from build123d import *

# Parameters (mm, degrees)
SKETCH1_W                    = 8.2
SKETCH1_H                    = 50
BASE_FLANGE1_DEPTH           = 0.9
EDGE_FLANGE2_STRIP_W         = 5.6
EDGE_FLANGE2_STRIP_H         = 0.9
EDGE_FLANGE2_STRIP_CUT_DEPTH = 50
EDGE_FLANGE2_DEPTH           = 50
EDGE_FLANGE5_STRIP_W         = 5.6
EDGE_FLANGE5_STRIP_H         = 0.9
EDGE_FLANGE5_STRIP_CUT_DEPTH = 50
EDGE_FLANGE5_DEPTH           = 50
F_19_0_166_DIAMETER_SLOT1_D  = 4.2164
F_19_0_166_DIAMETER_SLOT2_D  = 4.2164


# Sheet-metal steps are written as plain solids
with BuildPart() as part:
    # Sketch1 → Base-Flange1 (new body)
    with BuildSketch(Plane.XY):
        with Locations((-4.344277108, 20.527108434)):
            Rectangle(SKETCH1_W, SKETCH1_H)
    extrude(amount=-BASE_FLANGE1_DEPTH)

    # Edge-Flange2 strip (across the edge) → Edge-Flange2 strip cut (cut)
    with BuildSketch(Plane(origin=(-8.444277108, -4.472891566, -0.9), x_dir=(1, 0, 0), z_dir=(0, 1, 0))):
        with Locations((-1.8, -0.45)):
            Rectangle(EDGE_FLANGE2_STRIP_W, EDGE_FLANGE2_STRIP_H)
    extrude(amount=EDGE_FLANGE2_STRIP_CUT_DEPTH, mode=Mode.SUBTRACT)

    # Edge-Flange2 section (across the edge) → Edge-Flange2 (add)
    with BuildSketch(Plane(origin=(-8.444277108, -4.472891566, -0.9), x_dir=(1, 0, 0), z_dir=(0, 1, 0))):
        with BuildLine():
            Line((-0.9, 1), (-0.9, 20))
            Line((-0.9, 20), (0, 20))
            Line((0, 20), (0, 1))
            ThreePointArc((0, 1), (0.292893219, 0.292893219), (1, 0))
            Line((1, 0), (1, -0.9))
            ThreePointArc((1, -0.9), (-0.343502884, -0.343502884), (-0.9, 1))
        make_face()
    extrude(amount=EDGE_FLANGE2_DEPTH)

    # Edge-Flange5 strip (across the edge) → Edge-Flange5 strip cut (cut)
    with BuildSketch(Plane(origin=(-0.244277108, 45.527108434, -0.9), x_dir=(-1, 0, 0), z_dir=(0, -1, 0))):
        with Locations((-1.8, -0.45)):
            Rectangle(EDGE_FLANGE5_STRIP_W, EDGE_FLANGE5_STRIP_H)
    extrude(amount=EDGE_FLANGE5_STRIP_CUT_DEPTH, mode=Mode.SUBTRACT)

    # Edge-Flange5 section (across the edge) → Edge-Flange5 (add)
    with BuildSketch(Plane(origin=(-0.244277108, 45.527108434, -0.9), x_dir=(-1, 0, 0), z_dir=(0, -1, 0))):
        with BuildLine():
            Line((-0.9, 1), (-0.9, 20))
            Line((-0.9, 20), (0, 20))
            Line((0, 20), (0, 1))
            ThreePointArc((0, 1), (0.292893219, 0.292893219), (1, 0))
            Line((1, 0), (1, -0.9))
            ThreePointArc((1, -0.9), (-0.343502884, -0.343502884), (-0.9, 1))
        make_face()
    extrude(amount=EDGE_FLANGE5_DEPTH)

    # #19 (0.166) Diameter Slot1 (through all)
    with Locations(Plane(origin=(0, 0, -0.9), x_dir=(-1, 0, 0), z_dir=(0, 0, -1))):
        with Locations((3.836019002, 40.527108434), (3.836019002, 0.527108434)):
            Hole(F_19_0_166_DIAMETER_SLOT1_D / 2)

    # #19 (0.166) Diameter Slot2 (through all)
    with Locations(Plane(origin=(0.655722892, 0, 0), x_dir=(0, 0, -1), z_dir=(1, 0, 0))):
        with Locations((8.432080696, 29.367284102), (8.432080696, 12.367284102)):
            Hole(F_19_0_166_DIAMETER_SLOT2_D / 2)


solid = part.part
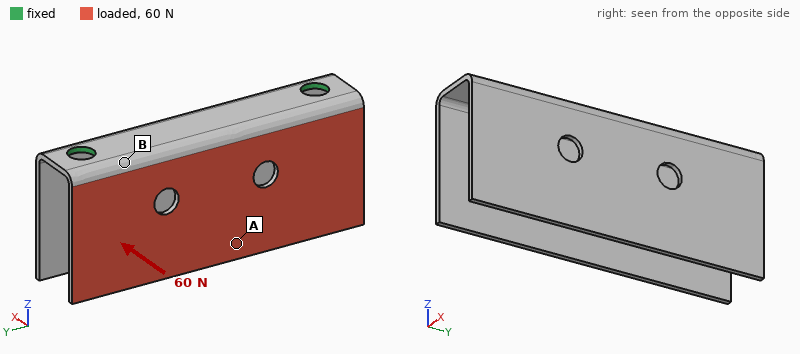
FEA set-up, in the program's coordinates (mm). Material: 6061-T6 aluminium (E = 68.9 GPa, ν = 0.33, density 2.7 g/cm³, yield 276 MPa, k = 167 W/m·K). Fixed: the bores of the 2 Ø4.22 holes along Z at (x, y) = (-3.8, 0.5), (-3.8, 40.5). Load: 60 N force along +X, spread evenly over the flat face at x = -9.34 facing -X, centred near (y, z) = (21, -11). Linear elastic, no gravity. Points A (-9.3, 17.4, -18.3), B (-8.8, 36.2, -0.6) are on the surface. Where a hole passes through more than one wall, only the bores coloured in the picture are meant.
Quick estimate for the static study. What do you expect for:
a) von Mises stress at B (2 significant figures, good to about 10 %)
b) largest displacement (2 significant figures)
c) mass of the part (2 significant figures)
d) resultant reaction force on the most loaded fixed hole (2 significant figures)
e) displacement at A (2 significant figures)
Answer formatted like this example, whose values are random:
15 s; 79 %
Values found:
80 MPa; 0.55 mm; 5.7 g; 30 N; 0.46 mm
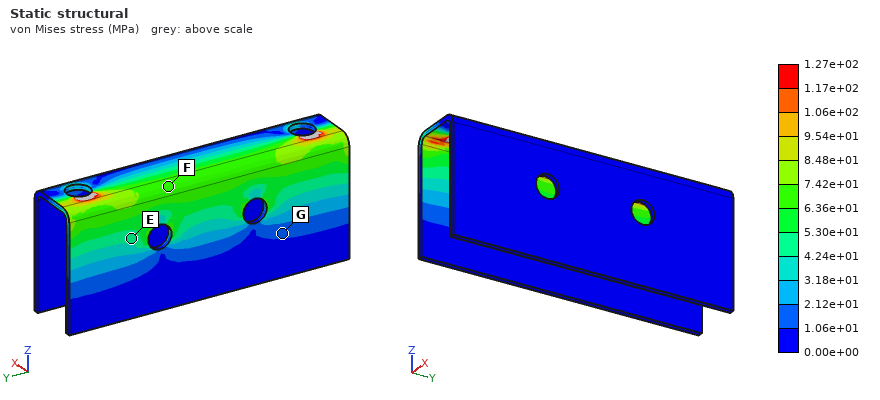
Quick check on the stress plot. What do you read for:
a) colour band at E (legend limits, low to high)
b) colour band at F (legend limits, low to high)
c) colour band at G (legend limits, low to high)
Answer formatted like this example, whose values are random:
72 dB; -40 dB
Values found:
4.24e+01 to 5.30e+01 MPa; 6.36e+01 to 7.42e+01 MPa; 1.06e+01 to 2.12e+01 MPa
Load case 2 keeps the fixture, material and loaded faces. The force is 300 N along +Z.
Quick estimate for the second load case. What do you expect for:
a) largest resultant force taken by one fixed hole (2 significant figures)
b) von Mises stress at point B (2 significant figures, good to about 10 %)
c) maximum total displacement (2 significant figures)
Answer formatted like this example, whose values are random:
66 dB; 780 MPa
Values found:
160 N; 50 MPa; 0.43 mm
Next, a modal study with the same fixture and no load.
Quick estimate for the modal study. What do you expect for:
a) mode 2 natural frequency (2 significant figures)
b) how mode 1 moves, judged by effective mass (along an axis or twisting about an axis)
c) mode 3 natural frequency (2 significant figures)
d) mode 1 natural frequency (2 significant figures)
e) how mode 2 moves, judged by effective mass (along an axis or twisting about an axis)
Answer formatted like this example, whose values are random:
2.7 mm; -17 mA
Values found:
1500 Hz; along X; 2100 Hz; 1400 Hz; along X
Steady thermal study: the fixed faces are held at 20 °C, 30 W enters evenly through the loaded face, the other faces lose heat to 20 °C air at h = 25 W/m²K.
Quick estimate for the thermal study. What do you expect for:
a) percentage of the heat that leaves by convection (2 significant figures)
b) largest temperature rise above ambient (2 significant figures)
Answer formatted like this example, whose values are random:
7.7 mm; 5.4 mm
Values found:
9.9 %; 78 K
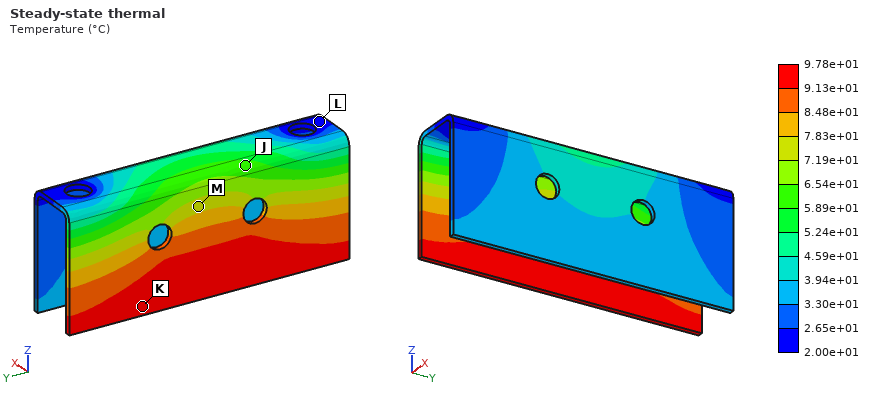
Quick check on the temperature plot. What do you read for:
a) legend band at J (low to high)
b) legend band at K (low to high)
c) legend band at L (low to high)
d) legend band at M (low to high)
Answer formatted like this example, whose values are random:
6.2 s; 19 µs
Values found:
5.89e+01 to 6.54e+01 °C; 9.13e+01 to 9.78e+01 °C; 2.00e+01 to 2.65e+01 °C; 7.19e+01 to 7.83e+01 °C
